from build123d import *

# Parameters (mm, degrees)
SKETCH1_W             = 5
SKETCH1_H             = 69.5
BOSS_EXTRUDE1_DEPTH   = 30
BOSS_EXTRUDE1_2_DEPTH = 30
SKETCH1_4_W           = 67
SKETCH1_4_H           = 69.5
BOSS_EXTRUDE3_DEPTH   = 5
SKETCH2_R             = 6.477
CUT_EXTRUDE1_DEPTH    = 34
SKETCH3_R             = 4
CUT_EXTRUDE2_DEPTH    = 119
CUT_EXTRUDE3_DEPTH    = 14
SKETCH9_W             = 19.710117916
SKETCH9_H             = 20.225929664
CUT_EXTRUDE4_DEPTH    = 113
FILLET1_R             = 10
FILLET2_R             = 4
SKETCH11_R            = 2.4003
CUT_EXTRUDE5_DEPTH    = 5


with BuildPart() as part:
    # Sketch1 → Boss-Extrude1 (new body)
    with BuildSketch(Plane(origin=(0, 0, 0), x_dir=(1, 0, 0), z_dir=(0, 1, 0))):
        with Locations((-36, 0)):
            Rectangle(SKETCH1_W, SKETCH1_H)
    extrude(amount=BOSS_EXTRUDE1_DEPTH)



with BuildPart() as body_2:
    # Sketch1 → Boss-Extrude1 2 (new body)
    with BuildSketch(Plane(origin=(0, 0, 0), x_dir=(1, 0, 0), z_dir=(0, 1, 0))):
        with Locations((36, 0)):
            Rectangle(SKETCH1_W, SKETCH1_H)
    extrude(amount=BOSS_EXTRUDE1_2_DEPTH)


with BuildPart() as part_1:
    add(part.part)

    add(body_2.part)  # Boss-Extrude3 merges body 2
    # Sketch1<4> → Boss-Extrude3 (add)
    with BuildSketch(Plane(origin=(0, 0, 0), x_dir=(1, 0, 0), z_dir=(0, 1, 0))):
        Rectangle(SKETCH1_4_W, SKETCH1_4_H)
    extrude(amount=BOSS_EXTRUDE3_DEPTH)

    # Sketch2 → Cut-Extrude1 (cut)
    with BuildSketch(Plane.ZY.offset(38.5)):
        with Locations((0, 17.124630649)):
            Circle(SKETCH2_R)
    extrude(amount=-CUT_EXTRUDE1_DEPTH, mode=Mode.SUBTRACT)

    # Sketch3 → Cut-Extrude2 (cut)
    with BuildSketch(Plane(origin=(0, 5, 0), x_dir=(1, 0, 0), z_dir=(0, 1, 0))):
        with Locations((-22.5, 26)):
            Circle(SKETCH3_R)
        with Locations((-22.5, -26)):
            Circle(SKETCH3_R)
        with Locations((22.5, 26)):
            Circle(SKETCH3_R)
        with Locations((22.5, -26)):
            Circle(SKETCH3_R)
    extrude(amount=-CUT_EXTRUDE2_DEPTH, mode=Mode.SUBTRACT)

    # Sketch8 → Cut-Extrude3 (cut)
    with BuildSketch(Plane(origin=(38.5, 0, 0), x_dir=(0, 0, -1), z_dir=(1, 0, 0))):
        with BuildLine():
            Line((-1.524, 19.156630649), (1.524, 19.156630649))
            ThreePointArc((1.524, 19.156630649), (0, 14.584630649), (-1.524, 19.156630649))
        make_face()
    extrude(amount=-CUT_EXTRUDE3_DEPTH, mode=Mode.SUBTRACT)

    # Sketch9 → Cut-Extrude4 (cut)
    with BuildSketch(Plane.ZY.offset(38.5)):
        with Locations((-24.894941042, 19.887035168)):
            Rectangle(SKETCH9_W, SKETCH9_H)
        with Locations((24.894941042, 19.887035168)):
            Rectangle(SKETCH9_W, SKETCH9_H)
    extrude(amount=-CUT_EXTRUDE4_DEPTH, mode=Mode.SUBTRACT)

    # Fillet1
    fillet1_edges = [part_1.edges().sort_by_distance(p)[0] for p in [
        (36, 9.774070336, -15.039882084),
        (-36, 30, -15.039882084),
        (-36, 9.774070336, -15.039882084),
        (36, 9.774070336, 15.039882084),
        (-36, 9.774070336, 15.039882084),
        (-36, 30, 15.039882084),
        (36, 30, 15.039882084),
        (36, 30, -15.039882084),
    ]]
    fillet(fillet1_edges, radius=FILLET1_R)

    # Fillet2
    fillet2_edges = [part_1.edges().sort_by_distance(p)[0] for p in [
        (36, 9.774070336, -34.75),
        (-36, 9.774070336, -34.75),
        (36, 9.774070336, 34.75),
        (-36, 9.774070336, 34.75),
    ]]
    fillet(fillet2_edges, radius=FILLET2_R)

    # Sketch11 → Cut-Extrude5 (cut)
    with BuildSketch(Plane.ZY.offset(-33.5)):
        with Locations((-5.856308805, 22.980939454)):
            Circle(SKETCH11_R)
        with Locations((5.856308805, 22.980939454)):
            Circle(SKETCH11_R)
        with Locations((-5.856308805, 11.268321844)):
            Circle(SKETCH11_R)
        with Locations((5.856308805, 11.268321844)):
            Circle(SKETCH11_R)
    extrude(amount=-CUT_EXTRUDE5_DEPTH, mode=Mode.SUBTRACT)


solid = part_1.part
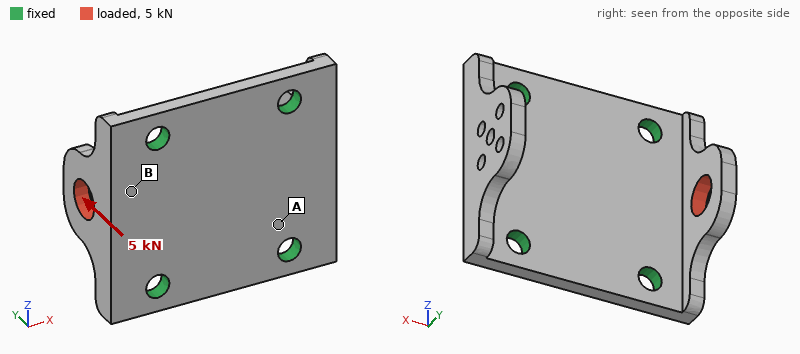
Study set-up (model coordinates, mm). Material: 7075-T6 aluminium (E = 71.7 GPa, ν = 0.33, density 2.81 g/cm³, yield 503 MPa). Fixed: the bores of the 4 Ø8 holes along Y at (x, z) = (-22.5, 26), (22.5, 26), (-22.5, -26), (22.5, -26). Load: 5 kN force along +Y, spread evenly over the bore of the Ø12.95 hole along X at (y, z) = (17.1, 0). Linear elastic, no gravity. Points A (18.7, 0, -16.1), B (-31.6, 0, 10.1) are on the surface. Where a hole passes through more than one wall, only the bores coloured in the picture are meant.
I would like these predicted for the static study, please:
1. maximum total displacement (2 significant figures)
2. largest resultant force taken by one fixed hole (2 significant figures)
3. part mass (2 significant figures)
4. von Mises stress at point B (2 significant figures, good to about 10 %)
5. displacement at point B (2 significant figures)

0.27 mm
2.8 kN
95 g
64 MPa
0.079 mm
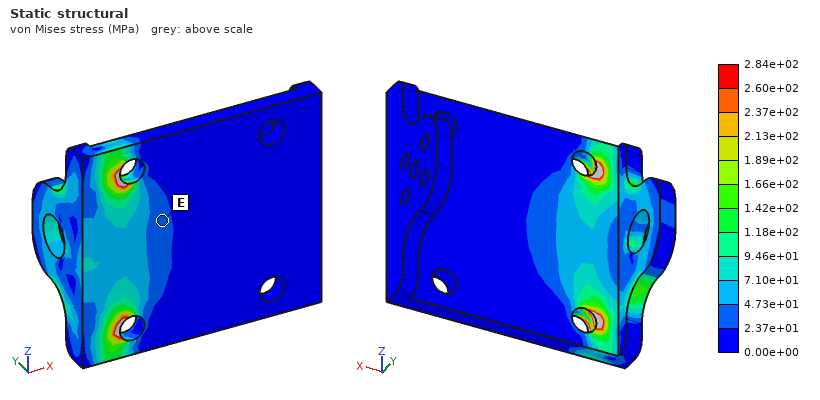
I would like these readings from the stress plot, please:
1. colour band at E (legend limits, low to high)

2.37e+01 to 4.73e+01 MPa
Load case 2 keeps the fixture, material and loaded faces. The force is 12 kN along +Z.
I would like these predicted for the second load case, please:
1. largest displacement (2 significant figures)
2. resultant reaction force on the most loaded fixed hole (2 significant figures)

0.21 mm
7.2 kN
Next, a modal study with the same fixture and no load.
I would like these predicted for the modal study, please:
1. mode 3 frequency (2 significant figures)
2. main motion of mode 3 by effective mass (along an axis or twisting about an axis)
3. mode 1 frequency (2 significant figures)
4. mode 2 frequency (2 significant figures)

9100 Hz
along Y
4500 Hz
4600 Hz
